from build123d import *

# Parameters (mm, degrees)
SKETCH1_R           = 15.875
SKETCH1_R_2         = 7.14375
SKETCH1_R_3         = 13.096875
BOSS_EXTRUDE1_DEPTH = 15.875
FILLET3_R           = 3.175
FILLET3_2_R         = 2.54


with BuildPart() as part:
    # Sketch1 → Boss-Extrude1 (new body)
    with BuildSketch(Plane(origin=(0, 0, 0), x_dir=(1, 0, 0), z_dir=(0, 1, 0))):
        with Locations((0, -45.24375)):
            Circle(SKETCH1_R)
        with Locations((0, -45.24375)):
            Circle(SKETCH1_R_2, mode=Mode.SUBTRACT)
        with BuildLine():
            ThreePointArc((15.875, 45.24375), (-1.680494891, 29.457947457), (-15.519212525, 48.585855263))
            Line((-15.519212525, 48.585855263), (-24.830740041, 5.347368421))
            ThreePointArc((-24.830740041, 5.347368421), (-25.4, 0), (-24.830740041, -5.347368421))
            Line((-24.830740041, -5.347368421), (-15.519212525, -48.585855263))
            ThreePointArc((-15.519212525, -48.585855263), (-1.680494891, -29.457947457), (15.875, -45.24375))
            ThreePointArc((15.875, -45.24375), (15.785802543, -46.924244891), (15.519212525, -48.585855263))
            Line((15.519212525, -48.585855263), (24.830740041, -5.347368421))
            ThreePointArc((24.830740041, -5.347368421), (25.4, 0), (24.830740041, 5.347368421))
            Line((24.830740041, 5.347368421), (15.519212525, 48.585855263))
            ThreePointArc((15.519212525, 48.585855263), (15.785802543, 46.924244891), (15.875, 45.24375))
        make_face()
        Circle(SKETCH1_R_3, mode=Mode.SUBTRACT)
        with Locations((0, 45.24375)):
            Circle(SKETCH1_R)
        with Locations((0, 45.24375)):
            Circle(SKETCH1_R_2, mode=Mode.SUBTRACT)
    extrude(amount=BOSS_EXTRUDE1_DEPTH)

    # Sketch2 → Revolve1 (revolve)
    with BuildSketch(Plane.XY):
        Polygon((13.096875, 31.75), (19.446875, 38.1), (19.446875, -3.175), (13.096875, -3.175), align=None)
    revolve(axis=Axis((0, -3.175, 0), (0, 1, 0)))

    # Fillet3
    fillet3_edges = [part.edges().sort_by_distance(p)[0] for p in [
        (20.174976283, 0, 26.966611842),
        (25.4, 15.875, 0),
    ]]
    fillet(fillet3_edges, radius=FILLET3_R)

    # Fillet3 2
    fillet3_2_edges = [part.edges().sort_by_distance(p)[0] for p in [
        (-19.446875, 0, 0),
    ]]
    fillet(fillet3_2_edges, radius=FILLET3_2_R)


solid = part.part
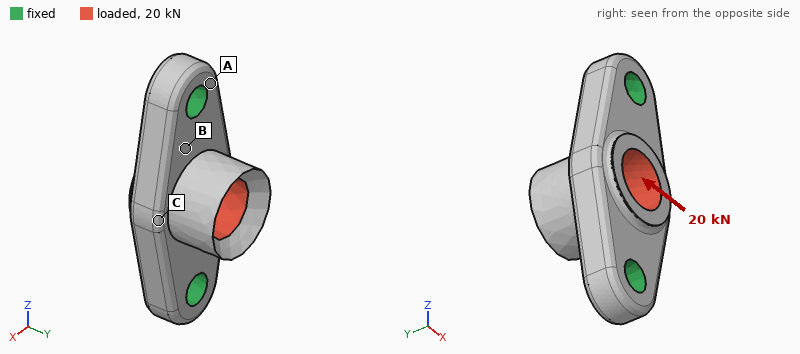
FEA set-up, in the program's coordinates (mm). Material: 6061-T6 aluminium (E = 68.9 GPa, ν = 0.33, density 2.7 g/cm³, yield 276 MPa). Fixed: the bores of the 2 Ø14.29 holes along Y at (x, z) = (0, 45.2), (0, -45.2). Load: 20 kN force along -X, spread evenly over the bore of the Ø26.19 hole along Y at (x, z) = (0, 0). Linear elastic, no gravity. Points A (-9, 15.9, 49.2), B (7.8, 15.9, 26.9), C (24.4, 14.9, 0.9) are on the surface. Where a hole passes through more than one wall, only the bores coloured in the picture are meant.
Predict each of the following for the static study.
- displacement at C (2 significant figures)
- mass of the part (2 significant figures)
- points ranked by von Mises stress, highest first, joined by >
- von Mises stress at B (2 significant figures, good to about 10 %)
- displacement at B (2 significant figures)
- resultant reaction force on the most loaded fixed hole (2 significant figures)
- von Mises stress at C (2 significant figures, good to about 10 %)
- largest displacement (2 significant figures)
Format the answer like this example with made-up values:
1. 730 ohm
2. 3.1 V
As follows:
1. 59 µm
2. 200 g
3. B > C > A
4. 64 MPa
5. 25 µm
6. 10 kN
7. 24 MPa
8. 95 µm
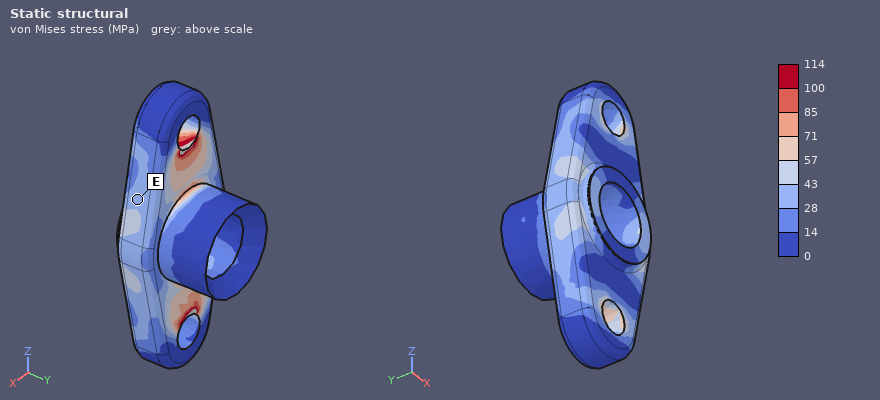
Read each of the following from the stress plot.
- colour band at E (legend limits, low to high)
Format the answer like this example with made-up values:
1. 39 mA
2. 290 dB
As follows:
1. 28 to 43 MPa
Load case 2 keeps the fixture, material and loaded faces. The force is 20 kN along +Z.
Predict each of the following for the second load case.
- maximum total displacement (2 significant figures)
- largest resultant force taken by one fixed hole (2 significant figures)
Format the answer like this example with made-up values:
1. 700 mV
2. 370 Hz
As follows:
1. 29 µm
2. 10 kN
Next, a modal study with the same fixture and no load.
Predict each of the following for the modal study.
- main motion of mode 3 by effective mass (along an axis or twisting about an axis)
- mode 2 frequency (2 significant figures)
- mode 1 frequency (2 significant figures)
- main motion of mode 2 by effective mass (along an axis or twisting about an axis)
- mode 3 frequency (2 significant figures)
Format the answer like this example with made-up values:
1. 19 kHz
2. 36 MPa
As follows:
1. along X
2. 8500 Hz
3. 7400 Hz
4. along Y
5. 13 kHz
